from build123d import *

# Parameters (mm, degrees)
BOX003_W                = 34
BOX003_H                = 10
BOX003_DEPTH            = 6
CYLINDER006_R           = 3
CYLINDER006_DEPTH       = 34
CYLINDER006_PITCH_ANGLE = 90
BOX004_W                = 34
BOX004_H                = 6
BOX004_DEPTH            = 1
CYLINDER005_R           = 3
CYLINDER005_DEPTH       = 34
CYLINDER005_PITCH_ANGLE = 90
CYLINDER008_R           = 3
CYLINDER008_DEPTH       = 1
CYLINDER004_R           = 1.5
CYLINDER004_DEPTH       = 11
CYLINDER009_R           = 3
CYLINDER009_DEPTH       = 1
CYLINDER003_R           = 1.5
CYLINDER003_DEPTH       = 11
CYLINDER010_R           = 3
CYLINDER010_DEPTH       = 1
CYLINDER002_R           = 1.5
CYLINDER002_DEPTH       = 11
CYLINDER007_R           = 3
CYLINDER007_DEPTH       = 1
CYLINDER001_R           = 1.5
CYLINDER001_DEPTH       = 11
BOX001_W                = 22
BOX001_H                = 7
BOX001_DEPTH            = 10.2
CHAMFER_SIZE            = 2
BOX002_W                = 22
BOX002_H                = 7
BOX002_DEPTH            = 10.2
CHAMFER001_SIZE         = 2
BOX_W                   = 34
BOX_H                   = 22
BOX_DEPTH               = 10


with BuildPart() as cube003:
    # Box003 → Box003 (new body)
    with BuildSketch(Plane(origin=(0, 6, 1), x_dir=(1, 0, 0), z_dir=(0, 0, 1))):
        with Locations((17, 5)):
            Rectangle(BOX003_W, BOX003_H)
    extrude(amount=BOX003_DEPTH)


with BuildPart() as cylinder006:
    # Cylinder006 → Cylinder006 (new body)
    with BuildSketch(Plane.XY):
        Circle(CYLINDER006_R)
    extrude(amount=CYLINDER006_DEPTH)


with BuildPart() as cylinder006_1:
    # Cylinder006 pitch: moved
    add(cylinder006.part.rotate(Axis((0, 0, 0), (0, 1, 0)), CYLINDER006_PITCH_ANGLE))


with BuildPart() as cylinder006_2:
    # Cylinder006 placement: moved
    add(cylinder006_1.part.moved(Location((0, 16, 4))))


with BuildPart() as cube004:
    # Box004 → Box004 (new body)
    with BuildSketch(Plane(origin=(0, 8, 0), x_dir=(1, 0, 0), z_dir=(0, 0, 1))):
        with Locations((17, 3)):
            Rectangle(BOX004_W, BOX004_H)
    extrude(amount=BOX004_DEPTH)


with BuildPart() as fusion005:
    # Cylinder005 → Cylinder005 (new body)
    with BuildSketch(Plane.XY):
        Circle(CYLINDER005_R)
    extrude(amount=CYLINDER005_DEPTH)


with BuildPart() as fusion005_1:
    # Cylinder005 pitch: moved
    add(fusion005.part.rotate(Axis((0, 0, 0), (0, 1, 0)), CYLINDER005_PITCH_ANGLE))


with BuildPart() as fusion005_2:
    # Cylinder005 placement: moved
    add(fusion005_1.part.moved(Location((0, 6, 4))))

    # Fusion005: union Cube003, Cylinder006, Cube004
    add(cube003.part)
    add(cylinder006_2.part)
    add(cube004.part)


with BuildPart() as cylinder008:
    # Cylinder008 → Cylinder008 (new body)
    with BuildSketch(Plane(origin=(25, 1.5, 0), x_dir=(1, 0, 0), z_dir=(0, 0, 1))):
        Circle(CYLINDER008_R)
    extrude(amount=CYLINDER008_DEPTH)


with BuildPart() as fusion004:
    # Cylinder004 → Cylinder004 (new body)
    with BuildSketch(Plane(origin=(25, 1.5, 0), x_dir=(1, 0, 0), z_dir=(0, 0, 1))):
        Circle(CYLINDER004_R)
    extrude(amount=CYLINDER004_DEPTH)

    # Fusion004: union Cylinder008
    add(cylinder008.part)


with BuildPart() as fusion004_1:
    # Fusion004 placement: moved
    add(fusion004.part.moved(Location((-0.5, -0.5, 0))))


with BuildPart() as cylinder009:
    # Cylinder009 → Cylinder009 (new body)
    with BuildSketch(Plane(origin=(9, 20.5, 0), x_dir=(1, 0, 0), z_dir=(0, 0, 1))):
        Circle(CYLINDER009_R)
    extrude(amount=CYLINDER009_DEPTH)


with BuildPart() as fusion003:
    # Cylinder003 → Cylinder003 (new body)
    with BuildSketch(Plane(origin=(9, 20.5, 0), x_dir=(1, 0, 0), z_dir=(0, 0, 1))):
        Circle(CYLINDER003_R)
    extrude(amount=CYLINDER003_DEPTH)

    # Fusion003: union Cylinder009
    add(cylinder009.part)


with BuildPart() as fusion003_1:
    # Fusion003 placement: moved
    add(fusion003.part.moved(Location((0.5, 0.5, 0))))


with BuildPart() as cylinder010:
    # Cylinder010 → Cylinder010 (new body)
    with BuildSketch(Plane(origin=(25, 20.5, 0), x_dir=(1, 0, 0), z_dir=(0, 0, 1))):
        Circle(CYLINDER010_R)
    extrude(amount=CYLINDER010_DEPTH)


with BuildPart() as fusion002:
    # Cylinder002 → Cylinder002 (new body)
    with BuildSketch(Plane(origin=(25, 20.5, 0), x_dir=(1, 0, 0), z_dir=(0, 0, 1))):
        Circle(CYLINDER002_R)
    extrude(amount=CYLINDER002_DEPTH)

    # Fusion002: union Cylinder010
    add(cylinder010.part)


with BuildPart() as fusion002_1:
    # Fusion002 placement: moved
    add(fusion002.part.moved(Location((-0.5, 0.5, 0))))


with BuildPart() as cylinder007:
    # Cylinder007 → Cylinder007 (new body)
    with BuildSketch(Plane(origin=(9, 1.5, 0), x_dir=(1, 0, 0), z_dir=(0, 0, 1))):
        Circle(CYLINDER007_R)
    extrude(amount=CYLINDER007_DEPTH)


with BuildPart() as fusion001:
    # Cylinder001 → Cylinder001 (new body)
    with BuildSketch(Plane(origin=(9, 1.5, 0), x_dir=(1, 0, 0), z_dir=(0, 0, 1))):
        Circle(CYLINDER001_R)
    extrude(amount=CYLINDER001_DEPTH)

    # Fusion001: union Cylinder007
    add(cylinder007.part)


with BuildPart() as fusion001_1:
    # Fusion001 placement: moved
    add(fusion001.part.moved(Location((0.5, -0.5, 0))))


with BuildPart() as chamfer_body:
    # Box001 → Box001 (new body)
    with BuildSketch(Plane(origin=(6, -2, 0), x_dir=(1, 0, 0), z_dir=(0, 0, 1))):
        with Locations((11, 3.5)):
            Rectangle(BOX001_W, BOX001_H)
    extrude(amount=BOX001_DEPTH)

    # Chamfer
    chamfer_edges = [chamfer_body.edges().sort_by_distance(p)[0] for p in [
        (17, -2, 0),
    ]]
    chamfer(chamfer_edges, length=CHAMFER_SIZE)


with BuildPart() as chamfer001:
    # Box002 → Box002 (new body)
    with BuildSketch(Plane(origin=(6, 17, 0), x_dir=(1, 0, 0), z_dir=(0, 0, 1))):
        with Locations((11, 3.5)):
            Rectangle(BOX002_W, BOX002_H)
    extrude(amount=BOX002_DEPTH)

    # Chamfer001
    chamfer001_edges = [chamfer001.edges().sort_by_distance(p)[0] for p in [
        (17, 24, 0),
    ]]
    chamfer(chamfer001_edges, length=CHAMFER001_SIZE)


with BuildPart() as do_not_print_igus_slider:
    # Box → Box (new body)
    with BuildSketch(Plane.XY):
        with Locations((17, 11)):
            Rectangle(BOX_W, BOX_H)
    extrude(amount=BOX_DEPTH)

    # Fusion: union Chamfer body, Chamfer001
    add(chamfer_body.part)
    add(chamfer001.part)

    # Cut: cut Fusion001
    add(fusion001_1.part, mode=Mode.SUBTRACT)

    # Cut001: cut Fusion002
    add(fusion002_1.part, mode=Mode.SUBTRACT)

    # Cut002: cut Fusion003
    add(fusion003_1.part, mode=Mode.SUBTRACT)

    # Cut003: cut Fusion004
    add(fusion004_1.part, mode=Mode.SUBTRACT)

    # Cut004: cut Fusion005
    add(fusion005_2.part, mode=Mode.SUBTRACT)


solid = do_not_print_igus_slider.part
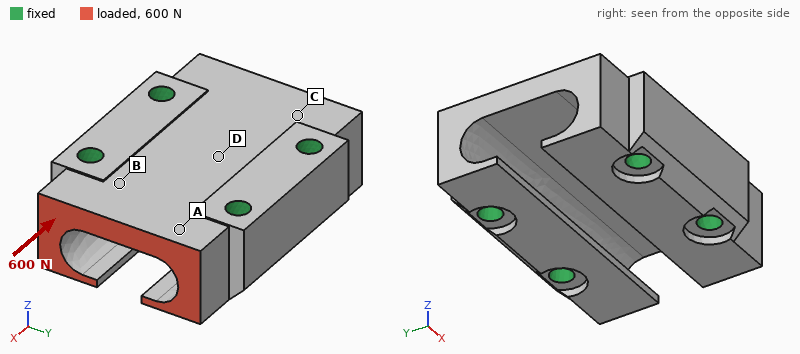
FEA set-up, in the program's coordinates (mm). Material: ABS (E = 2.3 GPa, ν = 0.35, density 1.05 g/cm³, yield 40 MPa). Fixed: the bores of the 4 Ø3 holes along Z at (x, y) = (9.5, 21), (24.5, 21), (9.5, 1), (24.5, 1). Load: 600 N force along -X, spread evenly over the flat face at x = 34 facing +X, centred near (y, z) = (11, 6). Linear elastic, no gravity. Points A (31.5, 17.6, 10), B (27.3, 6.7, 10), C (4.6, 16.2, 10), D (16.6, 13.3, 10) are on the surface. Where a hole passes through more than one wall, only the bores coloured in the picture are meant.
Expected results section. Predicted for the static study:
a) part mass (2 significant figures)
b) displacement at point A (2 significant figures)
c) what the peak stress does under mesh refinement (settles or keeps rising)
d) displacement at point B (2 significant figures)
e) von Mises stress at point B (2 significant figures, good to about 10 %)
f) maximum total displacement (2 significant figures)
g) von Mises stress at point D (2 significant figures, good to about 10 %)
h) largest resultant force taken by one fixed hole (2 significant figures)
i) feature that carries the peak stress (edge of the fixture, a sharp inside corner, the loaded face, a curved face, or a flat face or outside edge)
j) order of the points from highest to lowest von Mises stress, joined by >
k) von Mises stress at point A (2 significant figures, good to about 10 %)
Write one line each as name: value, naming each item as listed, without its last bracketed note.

part mass: 5.0 g
displacement at point A: 19 µm
what the peak stress does under mesh refinement: keeps rising
displacement at point B: 16 µm
von Mises stress at point B: 3.7 MPa
maximum total displacement: 39 µm
von Mises stress at point D: 1.7 MPa
largest resultant force taken by one fixed hole: 260 N
feature that carries the peak stress: edge of the fixture
order of the points from highest to lowest von Mises stress, joined by >: A > B > D > C
von Mises stress at point A: 4.9 MPa
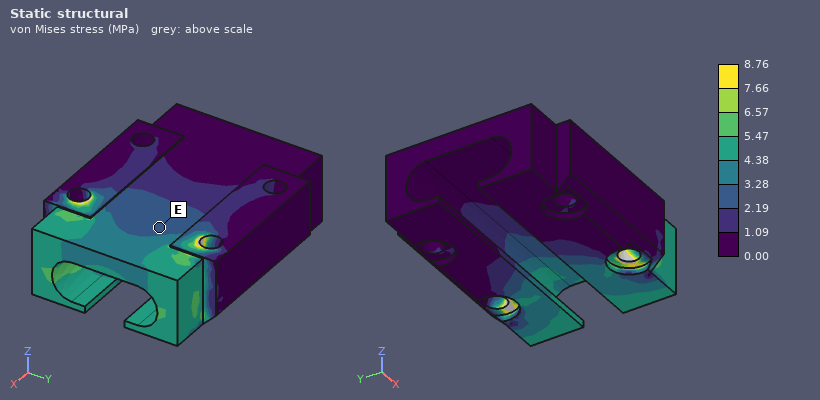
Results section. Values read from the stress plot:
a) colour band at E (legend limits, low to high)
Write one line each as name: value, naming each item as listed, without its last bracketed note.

colour band at E: 2.19 to 3.28 MPa
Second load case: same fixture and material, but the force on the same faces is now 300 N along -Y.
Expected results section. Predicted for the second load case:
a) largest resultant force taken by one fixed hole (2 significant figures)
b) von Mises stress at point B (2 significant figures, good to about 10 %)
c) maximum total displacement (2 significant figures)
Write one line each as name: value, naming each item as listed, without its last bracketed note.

largest resultant force taken by one fixed hole: 190 N
von Mises stress at point B: 5.7 MPa
maximum total displacement: 0.12 mm
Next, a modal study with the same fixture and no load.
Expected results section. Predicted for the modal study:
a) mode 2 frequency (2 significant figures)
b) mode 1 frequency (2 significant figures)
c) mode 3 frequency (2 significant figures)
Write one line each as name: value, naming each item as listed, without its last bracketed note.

mode 2 frequency: 11 kHz
mode 1 frequency: 11 kHz
mode 3 frequency: 12 kHz
